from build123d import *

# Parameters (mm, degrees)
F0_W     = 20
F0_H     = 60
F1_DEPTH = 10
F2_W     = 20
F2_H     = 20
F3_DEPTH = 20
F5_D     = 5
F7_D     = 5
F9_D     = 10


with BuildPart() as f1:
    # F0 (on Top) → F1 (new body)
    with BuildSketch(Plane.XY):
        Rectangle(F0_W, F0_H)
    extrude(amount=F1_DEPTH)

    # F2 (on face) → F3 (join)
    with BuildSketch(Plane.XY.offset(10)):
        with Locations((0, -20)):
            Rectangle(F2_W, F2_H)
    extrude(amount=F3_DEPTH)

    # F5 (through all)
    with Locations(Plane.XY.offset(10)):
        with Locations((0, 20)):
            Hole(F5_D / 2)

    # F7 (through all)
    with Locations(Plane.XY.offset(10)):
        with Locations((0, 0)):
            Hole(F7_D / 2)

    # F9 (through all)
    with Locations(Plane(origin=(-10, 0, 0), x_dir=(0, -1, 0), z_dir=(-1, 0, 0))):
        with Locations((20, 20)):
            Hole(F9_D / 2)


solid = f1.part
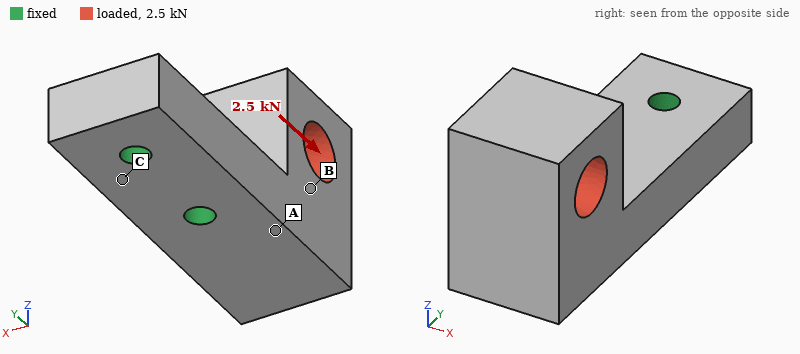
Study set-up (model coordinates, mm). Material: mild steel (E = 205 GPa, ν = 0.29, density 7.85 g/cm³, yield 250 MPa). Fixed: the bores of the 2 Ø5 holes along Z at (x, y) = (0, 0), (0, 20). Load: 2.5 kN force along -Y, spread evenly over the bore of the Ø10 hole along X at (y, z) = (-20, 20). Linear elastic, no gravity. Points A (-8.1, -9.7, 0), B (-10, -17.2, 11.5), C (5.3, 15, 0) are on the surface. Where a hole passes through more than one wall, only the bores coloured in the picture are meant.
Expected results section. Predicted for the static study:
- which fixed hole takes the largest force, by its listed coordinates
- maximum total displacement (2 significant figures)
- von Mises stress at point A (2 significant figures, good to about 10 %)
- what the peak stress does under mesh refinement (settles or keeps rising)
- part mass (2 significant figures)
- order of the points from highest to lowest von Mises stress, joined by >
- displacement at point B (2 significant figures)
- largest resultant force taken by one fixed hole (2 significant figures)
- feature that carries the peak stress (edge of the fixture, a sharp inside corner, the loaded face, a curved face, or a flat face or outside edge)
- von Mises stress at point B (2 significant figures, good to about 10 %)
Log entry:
(0, 0)
59 µm
84 MPa
keeps rising
140 g
A > B > C
20 µm
2.2 kN
edge of the fixture
39 MPa
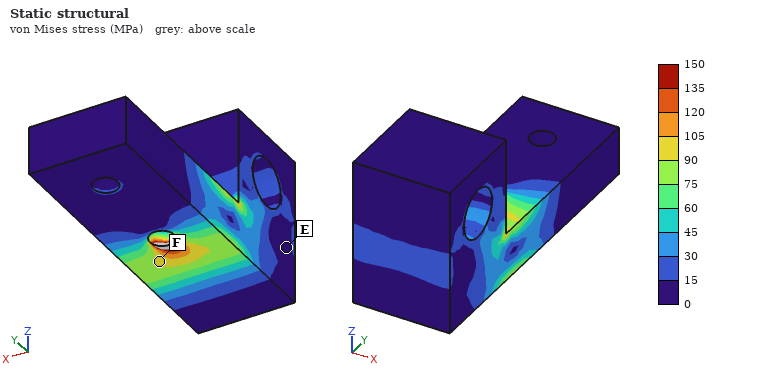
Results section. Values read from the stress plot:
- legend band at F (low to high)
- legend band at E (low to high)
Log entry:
90 to 105 MPa
0 to 15 MPa
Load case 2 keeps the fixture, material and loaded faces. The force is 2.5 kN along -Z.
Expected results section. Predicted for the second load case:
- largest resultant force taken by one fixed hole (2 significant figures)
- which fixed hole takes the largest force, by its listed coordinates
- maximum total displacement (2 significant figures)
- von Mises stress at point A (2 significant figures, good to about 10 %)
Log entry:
3.0 kN
(0, 0)
52 µm
66 MPa
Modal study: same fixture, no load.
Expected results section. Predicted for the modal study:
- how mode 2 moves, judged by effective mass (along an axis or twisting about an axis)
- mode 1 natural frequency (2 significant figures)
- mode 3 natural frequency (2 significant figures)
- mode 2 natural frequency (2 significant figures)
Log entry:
along X
4200 Hz
10 kHz
5500 Hz
